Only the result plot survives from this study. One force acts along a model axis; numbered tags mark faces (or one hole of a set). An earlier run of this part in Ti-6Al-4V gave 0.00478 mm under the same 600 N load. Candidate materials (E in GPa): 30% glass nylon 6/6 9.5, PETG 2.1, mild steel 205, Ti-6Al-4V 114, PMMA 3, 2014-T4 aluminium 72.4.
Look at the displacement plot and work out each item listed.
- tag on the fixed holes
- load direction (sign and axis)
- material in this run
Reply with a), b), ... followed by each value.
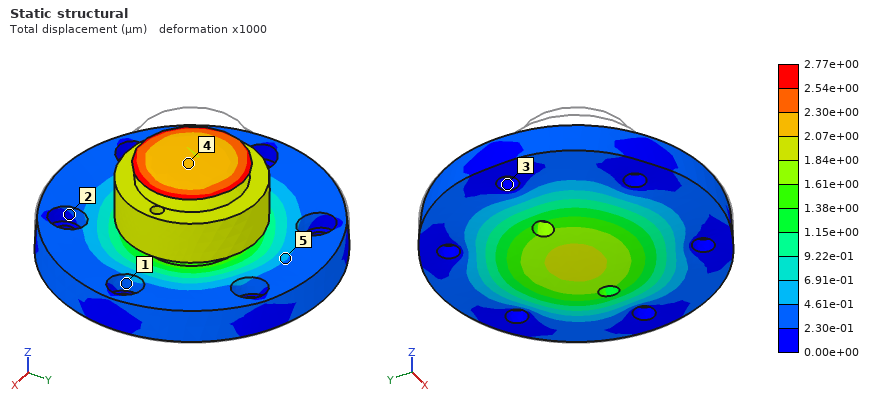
a) 3
b) -Z
c) mild steel
